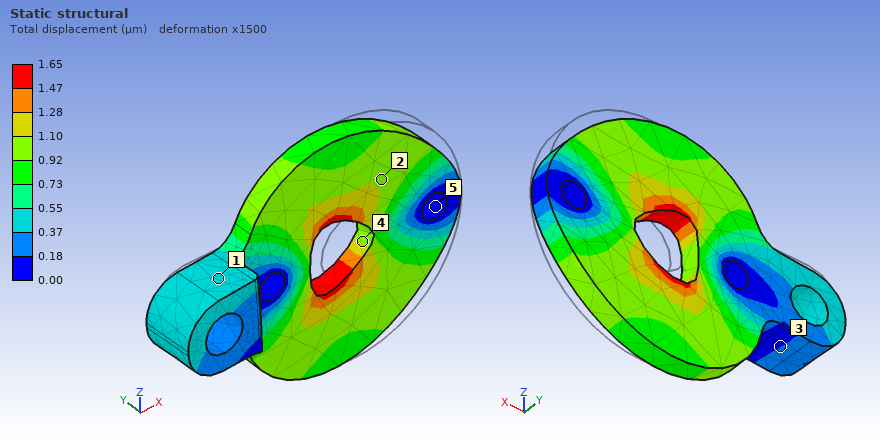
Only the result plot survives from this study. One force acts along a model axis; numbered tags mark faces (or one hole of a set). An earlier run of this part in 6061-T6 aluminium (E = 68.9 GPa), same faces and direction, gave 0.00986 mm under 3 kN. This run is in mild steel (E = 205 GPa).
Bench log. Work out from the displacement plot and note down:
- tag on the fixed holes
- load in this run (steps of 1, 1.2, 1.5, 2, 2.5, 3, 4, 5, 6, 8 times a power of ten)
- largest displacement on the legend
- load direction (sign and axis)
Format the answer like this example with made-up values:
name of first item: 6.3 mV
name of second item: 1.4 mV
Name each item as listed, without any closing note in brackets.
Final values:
tag on the fixed holes: 5
load in this run: 1.5 kN
largest displacement on the legend: 1.65 µm
load direction: -X
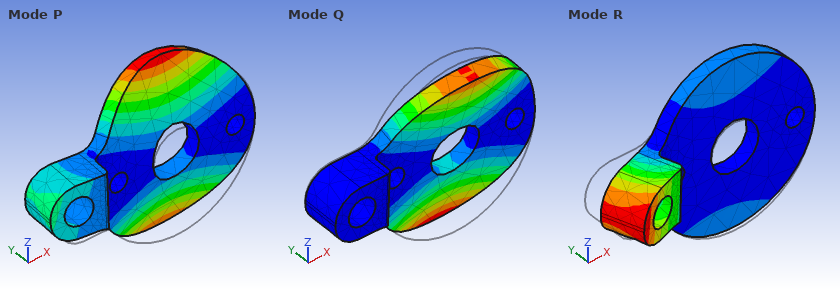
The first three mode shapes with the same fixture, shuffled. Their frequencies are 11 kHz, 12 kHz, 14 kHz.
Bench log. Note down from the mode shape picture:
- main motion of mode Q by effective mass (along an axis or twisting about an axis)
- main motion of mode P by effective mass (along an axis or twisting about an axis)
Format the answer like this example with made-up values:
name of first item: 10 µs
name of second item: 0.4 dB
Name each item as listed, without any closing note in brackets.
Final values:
main motion of mode Q by effective mass: twisting about X
main motion of mode P by effective mass: along Y
